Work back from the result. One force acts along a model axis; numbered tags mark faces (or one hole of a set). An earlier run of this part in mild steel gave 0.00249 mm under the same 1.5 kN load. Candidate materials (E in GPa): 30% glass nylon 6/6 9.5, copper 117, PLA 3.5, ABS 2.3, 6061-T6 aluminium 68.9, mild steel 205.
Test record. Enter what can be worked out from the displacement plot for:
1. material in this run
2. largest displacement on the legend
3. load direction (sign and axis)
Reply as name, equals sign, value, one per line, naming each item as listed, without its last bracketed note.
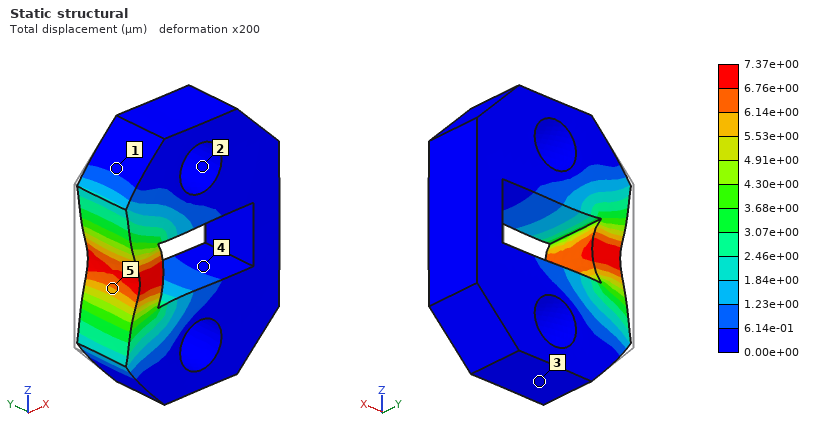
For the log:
material in this run = 6061-T6 aluminium
largest displacement on the legend = 7.37e+00 µm
load direction = +X
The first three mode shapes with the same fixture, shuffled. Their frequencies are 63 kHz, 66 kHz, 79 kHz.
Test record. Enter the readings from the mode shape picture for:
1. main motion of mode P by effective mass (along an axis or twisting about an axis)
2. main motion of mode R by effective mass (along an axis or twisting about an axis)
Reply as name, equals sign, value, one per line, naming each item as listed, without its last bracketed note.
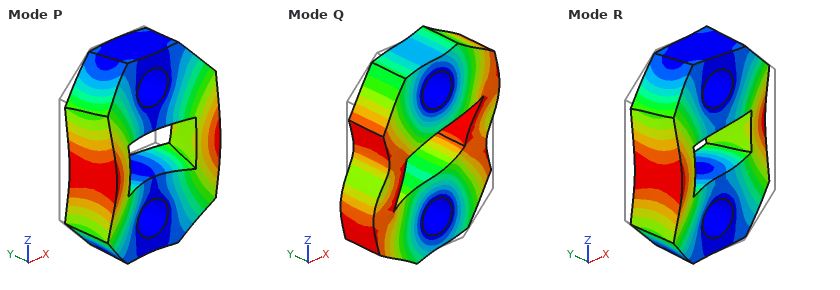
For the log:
main motion of mode P by effective mass = along Y
main motion of mode R by effective mass = twisting about Z
